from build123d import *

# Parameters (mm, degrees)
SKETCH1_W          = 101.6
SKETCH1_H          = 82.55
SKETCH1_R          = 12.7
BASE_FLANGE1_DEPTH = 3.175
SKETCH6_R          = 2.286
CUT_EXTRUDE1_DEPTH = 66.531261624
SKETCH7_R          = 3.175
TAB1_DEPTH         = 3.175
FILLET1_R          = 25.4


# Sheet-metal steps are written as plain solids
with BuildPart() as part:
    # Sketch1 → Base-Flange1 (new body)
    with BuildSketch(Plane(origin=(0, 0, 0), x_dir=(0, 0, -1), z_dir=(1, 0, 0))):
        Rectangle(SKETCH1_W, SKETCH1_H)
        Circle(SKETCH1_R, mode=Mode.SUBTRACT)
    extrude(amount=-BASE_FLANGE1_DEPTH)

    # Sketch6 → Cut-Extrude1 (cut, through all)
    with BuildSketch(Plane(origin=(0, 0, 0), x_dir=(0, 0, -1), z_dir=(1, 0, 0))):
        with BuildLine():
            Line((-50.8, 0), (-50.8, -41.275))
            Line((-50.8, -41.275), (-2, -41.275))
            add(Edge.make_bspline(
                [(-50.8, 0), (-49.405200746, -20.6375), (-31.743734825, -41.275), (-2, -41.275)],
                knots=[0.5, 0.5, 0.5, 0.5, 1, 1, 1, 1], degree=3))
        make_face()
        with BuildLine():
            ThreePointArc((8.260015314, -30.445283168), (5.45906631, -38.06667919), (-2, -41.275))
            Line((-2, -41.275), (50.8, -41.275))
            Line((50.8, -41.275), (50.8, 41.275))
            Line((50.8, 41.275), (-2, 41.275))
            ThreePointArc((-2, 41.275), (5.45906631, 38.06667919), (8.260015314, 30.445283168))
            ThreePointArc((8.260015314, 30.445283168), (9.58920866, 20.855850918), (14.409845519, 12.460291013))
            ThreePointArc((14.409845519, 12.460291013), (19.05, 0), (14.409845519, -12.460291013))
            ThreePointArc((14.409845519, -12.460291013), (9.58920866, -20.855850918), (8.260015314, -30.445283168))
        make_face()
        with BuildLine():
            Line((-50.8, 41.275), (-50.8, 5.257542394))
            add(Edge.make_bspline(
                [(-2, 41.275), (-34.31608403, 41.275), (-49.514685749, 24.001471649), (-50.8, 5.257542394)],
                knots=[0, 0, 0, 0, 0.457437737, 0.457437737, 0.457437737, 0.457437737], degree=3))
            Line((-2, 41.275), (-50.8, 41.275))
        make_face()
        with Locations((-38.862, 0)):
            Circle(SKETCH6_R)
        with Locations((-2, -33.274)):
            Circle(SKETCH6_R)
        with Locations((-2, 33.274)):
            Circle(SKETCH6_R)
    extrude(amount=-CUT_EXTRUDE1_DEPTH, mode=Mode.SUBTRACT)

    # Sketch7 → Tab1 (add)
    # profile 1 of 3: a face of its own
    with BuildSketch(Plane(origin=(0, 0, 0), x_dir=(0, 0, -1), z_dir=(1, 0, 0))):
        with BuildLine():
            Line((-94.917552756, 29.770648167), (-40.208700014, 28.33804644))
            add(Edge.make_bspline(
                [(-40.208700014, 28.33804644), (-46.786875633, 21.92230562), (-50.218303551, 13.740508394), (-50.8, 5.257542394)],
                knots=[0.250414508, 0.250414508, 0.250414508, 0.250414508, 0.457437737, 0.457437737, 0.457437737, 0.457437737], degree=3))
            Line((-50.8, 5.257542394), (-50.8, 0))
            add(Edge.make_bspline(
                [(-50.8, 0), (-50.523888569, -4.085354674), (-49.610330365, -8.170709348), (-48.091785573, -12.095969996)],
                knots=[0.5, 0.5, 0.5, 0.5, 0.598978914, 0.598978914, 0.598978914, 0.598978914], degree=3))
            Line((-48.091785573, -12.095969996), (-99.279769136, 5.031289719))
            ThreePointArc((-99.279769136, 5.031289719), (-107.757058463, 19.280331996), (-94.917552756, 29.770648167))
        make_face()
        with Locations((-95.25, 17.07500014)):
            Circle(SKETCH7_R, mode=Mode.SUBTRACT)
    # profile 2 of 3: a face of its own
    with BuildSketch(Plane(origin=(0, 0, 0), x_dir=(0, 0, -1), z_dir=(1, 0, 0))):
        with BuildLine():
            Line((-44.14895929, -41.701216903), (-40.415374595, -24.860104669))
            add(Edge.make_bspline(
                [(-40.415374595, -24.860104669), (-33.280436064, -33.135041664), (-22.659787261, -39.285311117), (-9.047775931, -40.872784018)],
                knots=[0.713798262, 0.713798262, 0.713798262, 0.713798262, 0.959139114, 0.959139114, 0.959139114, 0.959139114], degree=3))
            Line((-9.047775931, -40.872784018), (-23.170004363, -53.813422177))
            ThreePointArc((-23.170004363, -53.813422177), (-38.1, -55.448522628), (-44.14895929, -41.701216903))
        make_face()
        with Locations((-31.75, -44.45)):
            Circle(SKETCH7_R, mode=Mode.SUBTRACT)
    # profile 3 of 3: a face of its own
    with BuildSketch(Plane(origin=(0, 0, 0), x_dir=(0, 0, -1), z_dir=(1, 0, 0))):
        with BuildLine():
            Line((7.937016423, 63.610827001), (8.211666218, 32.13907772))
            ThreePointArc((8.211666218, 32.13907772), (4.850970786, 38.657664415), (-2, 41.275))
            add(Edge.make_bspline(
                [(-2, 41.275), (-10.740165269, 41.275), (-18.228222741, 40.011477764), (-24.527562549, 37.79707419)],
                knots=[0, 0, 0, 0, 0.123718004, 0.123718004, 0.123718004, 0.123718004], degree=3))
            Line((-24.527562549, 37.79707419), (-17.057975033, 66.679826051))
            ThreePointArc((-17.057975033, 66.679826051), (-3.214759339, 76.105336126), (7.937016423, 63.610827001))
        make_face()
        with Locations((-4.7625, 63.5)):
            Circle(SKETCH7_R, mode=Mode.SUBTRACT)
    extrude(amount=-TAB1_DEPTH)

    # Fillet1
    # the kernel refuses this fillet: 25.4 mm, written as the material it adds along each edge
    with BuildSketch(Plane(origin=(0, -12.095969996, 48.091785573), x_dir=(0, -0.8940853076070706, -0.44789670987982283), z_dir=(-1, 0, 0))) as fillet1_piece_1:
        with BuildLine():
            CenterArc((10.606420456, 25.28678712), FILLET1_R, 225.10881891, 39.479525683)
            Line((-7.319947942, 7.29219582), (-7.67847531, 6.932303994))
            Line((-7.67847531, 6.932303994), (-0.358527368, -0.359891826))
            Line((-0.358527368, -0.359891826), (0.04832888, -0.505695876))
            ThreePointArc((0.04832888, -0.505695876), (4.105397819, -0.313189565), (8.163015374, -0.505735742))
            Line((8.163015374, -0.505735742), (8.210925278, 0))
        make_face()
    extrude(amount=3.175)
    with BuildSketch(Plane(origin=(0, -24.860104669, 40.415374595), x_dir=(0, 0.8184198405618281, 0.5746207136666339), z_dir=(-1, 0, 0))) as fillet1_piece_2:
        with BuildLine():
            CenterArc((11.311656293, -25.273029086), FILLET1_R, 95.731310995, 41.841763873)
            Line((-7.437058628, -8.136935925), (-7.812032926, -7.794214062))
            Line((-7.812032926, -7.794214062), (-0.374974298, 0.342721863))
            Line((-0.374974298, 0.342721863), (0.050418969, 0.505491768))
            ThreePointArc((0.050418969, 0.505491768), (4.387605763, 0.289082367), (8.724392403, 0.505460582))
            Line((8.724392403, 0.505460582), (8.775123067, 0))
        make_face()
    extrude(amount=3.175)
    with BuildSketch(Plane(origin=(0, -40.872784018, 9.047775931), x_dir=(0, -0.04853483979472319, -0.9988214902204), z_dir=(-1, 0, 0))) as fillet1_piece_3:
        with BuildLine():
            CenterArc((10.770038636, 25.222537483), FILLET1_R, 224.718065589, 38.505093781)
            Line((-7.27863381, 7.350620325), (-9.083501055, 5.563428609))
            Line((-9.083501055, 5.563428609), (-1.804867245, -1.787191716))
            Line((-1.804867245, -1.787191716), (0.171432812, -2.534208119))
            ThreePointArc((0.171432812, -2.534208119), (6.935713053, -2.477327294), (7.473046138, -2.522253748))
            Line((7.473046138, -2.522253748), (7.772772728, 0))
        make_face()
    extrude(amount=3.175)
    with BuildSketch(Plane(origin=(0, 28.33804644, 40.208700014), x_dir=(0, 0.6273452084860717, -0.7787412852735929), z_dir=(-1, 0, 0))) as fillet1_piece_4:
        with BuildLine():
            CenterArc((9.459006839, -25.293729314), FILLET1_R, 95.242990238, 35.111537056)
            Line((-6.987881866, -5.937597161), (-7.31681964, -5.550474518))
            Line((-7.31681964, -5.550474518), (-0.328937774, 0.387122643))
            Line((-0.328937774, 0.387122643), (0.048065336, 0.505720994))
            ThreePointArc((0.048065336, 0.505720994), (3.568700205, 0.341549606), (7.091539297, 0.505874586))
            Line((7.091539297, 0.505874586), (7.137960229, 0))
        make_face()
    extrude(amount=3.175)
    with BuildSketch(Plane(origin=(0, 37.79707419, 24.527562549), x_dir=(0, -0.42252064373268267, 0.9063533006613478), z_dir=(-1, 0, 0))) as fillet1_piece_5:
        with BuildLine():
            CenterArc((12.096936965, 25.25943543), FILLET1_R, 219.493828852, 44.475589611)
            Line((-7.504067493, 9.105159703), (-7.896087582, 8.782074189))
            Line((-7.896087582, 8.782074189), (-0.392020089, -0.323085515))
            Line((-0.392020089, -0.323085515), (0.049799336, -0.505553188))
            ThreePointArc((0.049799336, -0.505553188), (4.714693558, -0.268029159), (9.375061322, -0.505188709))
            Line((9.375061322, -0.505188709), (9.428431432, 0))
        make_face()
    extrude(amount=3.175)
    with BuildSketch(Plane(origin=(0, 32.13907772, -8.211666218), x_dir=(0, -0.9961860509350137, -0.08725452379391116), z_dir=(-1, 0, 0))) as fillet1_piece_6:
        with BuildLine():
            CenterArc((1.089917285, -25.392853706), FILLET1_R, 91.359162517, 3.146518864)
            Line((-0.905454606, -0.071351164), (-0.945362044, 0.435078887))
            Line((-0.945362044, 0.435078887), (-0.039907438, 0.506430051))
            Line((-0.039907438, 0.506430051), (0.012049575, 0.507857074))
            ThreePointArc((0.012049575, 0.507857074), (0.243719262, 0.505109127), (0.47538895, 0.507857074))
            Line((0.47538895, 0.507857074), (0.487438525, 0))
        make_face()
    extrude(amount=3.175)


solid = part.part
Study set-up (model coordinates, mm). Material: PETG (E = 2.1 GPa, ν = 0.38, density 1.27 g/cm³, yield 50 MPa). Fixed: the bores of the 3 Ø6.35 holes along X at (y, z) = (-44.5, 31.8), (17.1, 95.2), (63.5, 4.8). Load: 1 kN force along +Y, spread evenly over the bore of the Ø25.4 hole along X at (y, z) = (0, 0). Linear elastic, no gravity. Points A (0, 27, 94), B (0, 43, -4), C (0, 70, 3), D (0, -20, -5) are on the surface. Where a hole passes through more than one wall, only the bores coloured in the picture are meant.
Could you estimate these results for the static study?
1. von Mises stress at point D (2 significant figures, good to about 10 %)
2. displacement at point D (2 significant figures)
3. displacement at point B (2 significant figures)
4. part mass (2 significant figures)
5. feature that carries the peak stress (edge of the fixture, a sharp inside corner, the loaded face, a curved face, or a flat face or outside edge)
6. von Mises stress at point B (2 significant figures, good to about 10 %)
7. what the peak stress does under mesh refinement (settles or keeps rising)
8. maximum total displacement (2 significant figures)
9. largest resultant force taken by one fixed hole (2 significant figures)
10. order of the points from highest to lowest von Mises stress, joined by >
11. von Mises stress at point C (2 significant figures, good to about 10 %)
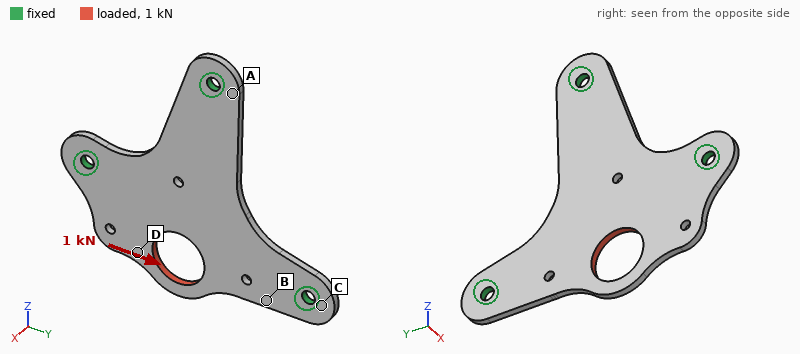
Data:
6.0 MPa
0.30 mm
0.077 mm
29 g
edge of the fixture
8.3 MPa
keeps rising
0.40 mm
550 N
B > D > C > A
3.0 MPa
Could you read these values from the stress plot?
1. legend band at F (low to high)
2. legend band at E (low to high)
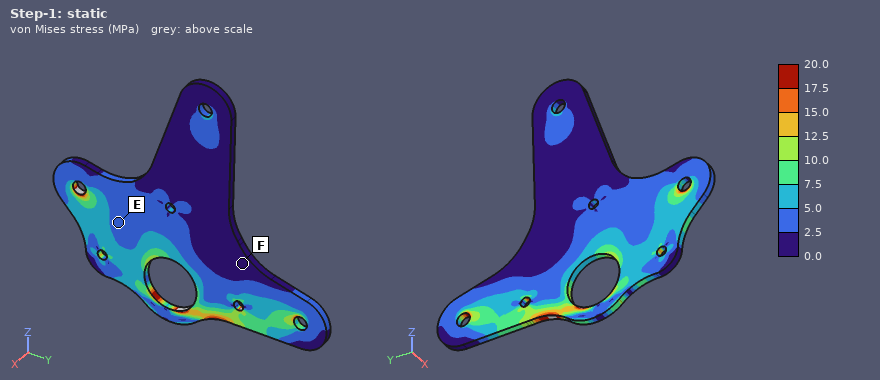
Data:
0.0 to 2.5 MPa
2.5 to 5.0 MPa
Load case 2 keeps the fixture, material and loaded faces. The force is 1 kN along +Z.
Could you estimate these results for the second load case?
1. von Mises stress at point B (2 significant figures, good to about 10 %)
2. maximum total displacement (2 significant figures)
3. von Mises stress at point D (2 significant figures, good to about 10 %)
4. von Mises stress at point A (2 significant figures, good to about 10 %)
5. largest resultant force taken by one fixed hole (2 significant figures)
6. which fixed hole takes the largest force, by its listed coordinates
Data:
2.5 MPa
0.36 mm
6.6 MPa
3.2 MPa
550 N
(17.1, 95.2)
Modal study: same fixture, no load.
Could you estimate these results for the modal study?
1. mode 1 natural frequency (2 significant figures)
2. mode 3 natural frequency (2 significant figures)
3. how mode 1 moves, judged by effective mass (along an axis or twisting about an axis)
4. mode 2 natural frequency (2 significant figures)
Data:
290 Hz
730 Hz
along X
440 Hz
